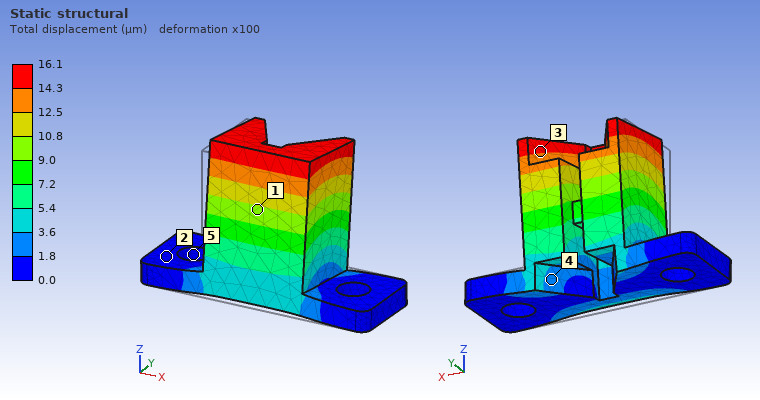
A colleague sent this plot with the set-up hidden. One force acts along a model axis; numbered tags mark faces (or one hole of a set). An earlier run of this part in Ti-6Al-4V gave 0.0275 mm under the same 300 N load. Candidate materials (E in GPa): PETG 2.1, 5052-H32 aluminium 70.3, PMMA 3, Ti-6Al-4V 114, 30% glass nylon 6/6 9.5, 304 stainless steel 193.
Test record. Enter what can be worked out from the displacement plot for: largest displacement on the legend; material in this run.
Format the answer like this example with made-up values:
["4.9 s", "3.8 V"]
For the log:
["16.1 µm", "304 stainless steel"]
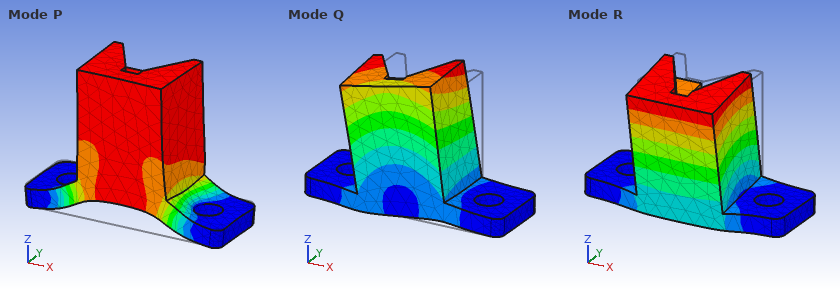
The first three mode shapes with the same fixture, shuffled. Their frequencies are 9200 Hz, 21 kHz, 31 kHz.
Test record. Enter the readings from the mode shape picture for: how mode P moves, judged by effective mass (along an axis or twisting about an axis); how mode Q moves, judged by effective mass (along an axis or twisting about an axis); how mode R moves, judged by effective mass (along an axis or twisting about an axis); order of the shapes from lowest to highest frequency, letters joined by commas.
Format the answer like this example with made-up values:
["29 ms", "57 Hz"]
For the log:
["along Z", "along X", "along Y", "R, Q, P"]
